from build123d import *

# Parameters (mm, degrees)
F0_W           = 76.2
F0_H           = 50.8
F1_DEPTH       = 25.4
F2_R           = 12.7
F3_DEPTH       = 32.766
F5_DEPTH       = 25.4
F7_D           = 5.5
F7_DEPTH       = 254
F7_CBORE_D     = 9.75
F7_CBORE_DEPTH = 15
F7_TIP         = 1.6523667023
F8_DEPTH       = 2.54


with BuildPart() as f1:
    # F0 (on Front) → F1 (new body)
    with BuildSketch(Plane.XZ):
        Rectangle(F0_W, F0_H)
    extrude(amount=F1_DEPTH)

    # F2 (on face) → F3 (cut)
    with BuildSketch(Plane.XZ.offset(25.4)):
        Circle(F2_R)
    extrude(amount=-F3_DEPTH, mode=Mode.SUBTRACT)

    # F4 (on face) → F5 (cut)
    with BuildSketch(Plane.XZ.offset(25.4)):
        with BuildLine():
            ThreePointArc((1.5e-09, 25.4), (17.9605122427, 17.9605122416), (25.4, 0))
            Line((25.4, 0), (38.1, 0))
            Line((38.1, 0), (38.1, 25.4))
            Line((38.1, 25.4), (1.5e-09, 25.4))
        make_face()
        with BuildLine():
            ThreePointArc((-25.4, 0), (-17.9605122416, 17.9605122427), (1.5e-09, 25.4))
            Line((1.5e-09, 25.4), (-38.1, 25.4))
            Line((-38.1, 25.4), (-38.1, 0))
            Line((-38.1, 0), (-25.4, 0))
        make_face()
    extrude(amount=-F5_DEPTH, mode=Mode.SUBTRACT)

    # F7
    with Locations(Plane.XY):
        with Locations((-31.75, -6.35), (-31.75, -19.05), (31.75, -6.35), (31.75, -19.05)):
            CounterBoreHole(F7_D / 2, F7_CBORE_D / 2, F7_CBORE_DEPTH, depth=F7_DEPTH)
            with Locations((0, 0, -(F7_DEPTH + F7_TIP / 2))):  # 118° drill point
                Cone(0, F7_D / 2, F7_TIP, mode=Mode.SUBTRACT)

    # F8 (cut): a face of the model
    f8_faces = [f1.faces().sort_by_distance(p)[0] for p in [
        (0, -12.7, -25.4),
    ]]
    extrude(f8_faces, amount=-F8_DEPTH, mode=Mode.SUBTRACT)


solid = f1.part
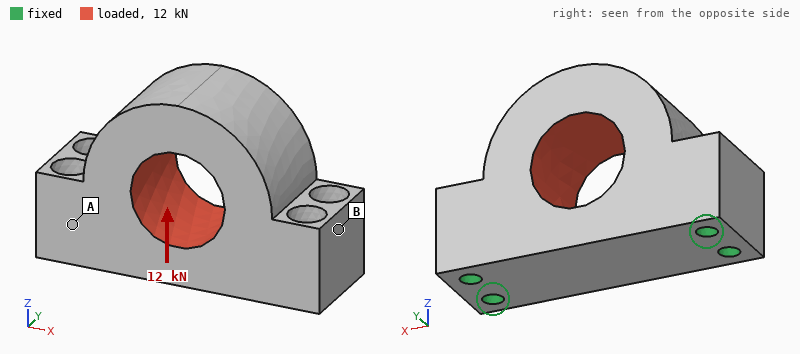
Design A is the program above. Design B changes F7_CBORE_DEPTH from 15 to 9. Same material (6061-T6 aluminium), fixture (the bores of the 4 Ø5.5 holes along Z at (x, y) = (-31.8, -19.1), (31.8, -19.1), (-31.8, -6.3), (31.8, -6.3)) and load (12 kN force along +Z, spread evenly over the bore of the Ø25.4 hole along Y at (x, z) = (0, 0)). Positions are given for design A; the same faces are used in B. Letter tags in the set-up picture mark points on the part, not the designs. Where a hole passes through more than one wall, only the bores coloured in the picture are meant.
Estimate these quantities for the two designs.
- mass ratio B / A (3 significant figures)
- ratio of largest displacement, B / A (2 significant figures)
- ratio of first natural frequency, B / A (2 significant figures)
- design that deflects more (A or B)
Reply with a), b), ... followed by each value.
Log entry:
a) 1.02
b) 0.75
c) 1.3
d) A
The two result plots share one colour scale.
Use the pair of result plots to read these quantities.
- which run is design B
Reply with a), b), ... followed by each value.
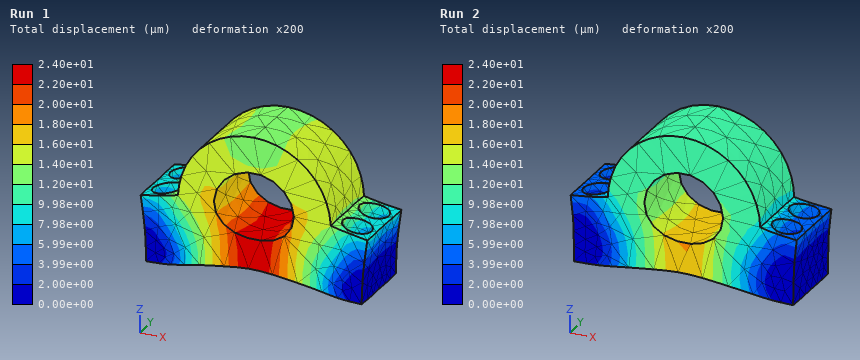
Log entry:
a) Run 2
